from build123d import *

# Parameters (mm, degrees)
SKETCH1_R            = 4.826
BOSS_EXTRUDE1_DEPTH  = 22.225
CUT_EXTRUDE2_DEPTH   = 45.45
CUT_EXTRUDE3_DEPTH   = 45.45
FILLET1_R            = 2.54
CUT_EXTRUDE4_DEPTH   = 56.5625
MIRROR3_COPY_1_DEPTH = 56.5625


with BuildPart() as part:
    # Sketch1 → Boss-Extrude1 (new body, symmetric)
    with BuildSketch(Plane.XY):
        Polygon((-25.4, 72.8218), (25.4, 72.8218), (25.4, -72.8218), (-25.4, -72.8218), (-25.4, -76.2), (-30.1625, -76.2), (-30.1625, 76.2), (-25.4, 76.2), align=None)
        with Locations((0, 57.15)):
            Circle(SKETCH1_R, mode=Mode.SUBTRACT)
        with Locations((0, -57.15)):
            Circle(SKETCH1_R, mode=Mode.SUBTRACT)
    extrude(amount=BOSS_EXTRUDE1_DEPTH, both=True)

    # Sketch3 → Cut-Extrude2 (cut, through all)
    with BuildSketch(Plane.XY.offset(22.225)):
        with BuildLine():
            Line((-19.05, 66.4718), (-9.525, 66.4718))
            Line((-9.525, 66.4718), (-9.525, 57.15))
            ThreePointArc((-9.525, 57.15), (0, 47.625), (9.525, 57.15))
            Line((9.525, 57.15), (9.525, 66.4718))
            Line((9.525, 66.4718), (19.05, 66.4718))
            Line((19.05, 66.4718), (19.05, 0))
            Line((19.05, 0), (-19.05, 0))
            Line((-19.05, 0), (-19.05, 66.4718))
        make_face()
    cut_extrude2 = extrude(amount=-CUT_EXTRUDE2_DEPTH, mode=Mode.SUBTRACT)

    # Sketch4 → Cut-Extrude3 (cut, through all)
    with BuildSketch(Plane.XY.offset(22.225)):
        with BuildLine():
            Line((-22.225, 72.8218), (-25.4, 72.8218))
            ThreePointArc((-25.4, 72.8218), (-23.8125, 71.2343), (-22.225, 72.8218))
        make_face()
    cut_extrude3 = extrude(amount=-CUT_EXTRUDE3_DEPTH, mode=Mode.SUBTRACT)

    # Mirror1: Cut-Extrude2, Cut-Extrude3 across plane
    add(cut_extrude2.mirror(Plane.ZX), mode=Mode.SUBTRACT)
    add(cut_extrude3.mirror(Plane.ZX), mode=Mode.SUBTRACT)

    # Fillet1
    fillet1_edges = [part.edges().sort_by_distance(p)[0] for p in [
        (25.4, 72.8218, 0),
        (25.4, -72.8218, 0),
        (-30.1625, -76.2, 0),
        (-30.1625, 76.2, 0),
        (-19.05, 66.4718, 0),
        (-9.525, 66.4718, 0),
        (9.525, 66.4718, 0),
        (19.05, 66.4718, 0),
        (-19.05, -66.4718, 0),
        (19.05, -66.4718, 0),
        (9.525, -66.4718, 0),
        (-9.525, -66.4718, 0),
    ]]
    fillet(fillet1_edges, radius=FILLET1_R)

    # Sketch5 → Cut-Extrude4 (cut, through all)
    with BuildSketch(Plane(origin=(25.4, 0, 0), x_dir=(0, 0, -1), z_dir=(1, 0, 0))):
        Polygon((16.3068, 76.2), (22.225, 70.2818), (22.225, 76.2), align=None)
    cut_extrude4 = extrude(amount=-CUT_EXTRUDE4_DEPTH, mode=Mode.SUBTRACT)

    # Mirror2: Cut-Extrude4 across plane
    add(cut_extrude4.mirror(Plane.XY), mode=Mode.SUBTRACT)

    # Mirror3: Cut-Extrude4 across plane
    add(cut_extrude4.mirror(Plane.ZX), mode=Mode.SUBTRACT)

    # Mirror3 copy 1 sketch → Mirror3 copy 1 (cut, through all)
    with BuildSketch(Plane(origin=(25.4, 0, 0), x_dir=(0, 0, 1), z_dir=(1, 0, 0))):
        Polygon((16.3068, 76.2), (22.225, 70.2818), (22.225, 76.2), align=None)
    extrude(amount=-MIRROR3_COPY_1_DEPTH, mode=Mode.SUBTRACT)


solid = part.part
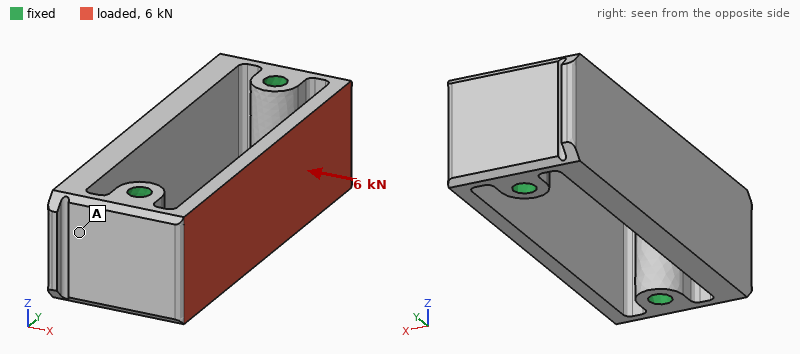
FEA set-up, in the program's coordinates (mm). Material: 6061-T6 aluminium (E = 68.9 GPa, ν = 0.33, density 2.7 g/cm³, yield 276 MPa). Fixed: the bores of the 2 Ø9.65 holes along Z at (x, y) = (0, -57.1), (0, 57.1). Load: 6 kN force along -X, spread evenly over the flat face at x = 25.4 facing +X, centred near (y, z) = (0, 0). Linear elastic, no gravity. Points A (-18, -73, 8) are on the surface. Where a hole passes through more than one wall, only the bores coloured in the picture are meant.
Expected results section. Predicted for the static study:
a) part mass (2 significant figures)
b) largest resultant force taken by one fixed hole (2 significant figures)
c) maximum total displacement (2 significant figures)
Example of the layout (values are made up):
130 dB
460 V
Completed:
420 g
5.8 kN
0.73 mm
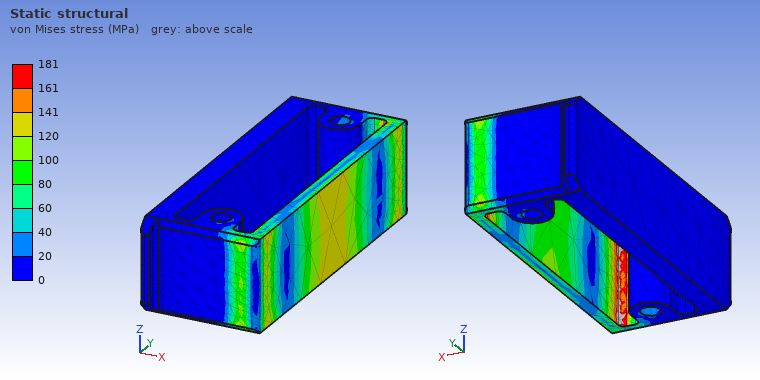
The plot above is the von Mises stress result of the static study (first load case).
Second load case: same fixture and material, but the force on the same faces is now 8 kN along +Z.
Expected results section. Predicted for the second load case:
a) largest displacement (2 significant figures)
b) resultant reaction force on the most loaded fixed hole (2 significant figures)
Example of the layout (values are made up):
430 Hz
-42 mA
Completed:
0.14 mm
4.0 kN
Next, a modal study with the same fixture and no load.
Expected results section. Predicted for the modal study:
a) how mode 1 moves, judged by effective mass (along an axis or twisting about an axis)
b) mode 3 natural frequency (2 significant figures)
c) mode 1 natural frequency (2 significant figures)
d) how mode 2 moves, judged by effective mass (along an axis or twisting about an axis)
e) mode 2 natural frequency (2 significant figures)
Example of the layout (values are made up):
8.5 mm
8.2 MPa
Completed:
along X
3500 Hz
1600 Hz
along X
2200 Hz
